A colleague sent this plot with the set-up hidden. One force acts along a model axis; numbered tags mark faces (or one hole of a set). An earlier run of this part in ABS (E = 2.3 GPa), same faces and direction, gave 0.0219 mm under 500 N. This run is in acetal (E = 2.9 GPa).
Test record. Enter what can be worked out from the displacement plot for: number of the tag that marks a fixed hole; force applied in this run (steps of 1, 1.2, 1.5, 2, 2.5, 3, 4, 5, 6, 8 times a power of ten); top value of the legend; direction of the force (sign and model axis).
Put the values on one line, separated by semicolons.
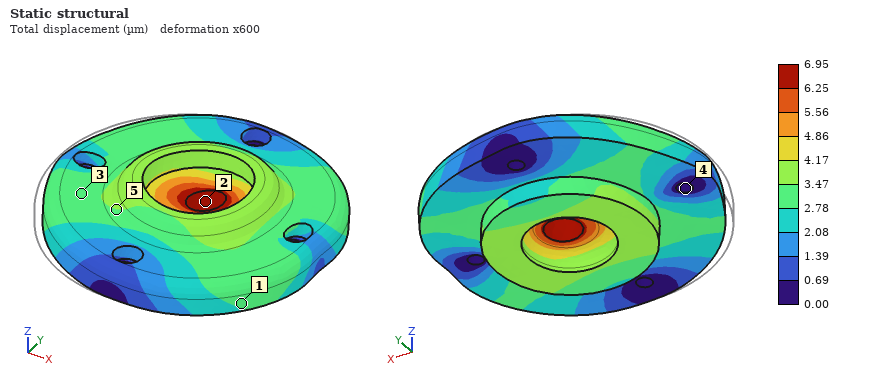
4; 200 N; 6.95 µm; +X
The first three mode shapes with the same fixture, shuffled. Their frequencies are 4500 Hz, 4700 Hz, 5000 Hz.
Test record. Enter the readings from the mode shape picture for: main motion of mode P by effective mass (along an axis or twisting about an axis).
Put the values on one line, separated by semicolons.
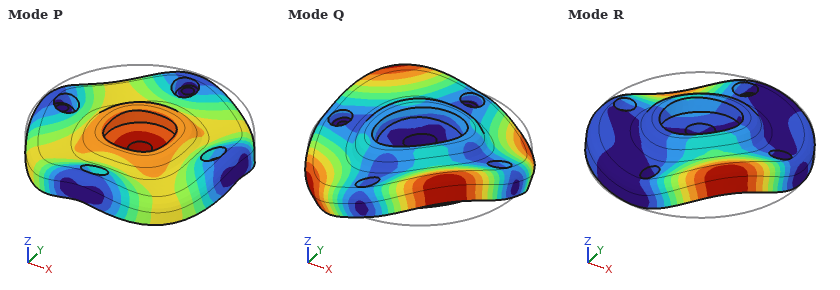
along Z
